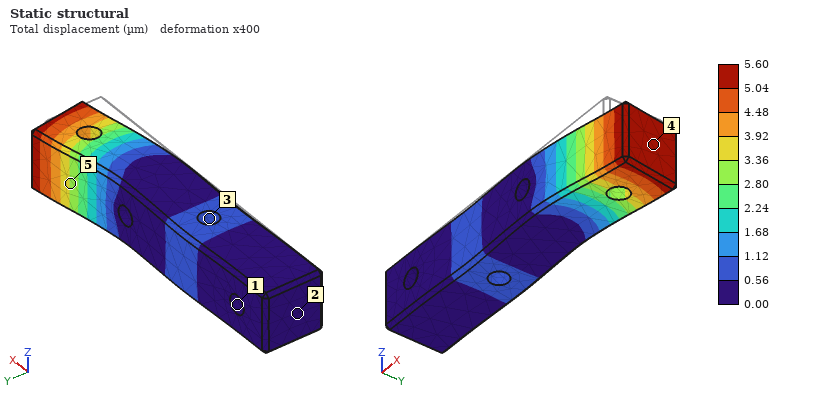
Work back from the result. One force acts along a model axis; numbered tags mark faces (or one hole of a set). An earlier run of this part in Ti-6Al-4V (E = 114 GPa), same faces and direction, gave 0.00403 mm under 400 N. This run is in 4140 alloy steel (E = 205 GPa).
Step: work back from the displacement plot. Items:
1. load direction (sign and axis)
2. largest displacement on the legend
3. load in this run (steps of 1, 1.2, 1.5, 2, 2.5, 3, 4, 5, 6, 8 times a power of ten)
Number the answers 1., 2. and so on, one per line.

1. +Y
2. 5.60 µm
3. 1 kN
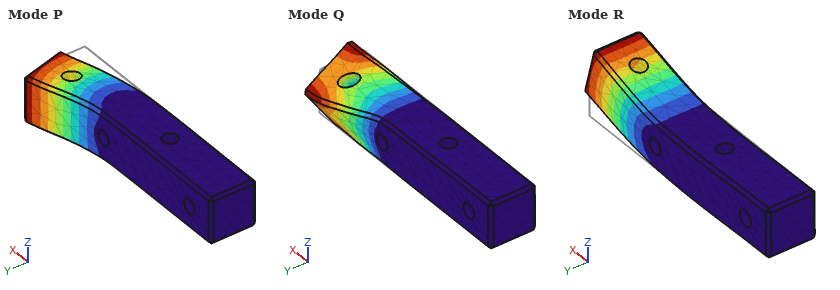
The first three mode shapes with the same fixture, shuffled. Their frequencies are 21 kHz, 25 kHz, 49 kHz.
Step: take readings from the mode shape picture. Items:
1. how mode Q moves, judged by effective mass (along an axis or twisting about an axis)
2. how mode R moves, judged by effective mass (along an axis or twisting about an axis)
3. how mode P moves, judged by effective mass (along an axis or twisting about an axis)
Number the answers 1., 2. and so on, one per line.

1. twisting about X
2. along Z
3. along Y
